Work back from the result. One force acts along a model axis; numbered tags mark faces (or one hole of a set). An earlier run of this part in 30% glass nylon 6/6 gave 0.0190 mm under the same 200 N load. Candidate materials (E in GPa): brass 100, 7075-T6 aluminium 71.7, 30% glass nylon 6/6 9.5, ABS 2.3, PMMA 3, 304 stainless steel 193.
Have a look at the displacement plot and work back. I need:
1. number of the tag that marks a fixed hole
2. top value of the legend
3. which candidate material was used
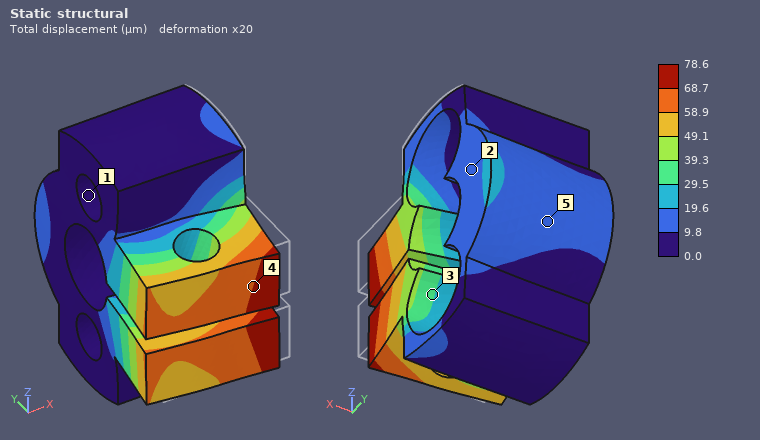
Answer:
1
78.6 µm
ABS
